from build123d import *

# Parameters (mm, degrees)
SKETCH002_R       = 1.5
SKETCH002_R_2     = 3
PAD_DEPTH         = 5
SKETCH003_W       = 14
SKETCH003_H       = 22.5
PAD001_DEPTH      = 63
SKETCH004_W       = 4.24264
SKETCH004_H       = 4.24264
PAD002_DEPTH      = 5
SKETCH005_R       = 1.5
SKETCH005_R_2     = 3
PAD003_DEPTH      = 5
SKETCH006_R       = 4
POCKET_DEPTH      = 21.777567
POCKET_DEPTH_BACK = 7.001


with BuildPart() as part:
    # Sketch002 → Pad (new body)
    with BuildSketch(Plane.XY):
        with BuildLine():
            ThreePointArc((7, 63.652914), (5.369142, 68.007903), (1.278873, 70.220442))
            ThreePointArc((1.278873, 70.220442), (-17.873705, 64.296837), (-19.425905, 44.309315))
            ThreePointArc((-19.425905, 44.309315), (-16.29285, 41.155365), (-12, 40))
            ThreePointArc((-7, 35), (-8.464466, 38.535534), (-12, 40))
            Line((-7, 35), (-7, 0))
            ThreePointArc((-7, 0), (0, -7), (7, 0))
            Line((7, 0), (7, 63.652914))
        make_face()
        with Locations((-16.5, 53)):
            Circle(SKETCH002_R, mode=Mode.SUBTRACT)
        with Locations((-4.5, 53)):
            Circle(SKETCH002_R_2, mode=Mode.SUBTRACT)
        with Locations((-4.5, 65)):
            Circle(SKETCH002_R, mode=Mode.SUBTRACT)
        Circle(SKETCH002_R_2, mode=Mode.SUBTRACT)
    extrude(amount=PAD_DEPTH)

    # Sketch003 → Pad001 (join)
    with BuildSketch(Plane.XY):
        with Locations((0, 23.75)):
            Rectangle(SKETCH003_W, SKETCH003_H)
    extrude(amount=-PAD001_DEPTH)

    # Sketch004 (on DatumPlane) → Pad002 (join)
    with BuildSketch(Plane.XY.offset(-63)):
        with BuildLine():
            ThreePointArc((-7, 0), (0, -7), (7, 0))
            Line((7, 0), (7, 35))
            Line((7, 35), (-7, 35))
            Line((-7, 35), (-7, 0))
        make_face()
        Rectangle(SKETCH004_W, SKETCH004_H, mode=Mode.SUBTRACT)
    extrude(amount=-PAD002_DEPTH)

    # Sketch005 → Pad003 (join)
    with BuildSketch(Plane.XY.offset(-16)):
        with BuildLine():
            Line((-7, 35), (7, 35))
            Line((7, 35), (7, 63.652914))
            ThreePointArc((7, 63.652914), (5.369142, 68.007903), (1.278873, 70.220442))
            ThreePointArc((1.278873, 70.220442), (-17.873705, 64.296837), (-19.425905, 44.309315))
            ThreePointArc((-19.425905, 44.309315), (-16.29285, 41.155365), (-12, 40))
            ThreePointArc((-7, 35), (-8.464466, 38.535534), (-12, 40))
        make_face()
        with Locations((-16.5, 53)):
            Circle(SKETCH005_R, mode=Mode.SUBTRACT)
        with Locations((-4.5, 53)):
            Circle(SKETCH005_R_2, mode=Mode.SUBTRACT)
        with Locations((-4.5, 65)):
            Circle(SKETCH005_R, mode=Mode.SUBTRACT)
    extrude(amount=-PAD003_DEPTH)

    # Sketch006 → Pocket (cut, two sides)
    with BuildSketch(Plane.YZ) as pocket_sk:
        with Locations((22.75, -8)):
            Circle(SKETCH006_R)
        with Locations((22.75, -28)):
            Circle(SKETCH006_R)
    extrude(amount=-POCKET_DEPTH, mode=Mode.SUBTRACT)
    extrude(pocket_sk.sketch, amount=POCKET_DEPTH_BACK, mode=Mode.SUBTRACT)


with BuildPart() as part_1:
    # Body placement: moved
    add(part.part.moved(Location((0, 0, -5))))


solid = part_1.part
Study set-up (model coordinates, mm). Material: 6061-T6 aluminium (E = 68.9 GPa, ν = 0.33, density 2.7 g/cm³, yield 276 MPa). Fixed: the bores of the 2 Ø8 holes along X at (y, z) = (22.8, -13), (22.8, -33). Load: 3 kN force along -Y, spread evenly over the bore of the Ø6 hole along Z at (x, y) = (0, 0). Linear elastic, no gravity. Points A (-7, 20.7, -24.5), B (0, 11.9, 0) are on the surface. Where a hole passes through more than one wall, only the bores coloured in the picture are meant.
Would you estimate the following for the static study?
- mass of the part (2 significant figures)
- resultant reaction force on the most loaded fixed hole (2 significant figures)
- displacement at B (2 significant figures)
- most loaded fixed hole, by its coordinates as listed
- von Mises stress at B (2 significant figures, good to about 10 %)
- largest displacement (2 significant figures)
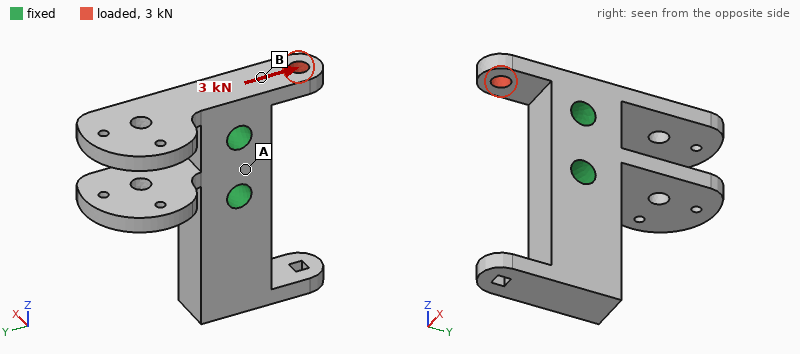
86 g
3.5 kN
15 µm
(22.8, -13)
45 MPa
39 µm
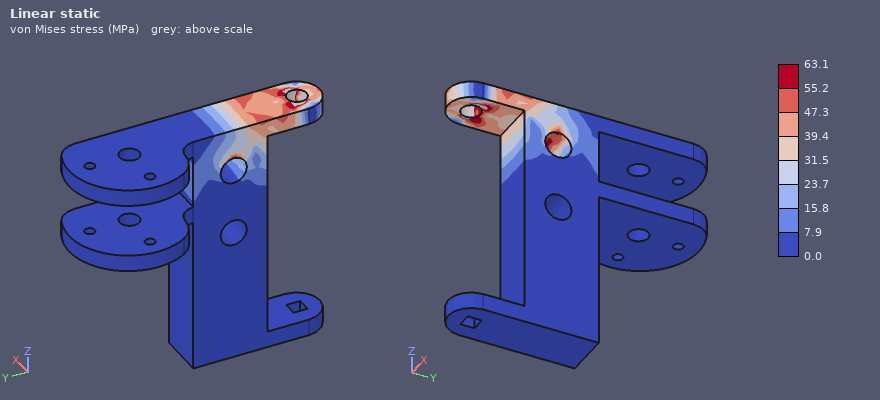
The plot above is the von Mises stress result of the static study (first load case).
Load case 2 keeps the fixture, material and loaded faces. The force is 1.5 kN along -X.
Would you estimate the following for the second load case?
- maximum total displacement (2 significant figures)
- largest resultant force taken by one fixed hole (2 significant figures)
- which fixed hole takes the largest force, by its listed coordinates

0.11 mm
1.5 kN
(22.8, -13)
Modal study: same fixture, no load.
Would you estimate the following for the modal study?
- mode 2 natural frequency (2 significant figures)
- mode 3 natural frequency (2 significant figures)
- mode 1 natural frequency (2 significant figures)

2400 Hz
4300 Hz
2200 Hz
